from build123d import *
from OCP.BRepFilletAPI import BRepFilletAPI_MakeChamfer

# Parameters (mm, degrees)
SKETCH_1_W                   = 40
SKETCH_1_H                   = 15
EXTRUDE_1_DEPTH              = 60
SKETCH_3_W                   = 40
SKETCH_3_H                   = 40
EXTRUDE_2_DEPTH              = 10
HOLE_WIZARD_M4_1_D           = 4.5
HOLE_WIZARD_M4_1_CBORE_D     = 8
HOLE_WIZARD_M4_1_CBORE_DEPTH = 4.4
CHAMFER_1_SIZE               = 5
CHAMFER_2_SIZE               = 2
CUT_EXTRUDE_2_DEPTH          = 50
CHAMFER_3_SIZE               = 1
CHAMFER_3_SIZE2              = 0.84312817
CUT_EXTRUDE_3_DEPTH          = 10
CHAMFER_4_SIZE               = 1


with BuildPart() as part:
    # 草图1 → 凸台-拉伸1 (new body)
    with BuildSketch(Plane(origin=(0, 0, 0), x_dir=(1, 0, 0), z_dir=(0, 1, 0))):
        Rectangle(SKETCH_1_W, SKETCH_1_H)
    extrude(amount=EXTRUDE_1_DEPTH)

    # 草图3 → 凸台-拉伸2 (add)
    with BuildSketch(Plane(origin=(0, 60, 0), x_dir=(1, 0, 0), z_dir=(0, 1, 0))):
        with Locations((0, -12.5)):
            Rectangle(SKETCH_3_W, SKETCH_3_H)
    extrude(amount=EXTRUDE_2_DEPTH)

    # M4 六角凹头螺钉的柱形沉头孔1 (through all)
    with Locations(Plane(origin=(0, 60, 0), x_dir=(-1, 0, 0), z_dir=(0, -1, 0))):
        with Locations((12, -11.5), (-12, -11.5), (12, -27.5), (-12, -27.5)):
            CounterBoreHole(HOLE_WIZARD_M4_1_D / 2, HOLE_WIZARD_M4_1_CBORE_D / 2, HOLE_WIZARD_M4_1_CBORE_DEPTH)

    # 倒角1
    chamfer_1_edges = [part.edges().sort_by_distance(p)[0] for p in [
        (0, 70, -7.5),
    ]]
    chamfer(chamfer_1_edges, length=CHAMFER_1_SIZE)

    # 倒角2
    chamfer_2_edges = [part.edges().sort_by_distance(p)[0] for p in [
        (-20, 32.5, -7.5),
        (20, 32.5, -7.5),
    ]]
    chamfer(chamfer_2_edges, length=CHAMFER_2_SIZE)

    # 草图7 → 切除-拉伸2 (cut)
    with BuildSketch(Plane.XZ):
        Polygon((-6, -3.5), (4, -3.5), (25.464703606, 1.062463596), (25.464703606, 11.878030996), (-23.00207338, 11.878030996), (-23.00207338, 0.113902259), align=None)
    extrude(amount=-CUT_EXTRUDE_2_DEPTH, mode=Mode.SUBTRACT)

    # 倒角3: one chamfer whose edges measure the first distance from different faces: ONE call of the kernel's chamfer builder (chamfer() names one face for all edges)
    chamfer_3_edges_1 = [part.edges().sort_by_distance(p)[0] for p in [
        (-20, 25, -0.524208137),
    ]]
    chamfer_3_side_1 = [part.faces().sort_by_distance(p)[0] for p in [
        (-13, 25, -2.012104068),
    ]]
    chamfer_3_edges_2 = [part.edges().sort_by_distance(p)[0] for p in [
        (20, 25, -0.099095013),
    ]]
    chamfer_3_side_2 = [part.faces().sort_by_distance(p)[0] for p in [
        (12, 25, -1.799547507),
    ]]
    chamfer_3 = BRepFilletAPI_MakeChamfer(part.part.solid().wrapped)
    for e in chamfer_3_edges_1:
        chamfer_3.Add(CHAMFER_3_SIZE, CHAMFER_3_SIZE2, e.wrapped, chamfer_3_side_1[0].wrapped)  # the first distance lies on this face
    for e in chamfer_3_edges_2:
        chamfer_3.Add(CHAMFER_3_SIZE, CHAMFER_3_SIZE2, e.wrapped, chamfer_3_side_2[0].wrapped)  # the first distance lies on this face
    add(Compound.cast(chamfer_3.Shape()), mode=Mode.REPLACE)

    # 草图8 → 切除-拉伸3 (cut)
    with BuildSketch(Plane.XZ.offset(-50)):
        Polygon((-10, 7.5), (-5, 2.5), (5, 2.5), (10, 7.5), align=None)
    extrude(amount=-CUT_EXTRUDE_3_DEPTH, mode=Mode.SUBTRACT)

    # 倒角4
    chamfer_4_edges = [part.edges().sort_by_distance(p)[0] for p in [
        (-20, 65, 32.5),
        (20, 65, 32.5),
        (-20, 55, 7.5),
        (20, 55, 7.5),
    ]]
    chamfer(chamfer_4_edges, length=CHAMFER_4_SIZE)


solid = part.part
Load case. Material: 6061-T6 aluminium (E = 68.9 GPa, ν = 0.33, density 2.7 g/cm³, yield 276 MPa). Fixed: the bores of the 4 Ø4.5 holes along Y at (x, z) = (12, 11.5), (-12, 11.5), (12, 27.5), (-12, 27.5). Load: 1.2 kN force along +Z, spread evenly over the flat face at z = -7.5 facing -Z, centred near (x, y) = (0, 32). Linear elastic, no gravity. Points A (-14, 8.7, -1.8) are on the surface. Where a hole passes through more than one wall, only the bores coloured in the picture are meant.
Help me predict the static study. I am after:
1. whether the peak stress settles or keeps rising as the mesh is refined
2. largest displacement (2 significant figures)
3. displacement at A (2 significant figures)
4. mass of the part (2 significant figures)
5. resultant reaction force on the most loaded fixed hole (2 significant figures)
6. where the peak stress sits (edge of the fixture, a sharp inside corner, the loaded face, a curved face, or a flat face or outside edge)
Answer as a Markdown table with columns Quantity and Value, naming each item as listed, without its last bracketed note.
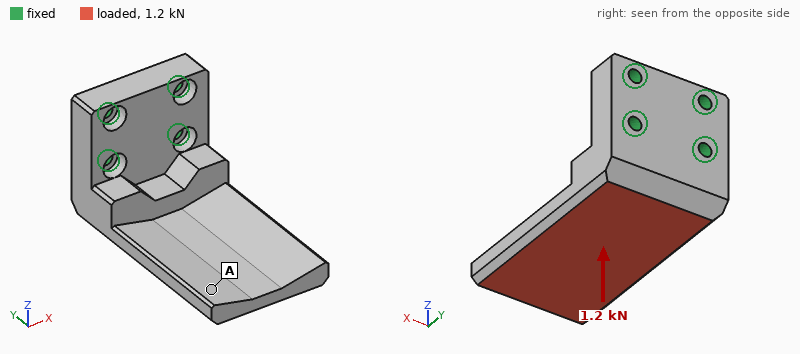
| Quantity | Value |
|---|---|
| whether the peak stress settles or keeps rising as the mesh is refined | keeps rising |
| largest displacement | 0.69 mm |
| displacement at A | 0.55 mm |
| mass of the part | 80 g |
| resultant reaction force on the most loaded fixed hole | 1.2 kN |
| where the peak stress sits | edge of the fixture |
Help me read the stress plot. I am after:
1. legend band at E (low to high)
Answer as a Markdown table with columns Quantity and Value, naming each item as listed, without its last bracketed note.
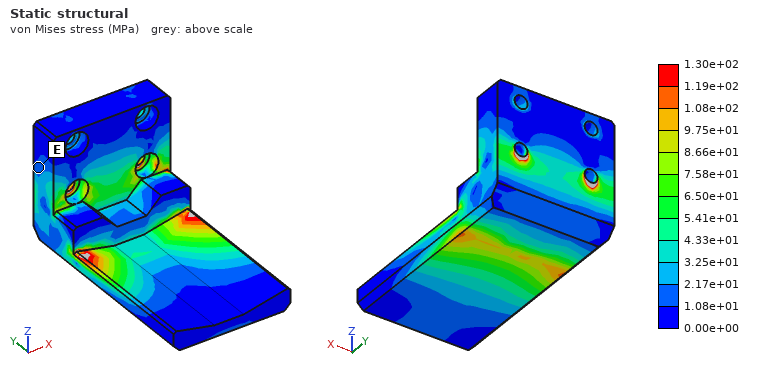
| Quantity | Value |
|---|---|
| legend band at E | 1.08e+01 to 2.17e+01 MPa |
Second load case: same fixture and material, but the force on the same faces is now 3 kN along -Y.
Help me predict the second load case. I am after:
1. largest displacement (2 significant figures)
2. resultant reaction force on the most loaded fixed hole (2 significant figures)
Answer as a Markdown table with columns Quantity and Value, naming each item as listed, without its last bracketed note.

| Quantity | Value |
|---|---|
| largest displacement | 0.41 mm |
| resultant reaction force on the most loaded fixed hole | 2.7 kN |
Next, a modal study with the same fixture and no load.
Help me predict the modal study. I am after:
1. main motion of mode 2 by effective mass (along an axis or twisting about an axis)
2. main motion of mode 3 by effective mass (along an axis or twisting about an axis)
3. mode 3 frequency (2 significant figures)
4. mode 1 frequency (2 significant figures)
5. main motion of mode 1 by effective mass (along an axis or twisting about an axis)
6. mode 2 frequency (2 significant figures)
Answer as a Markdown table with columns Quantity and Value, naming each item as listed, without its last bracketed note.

| Quantity | Value |
|---|---|
| main motion of mode 2 by effective mass | along X |
| main motion of mode 3 by effective mass | along X |
| mode 3 frequency | 4600 Hz |
| mode 1 frequency | 1400 Hz |
| main motion of mode 1 by effective mass | along Z |
| mode 2 frequency | 3500 Hz |
